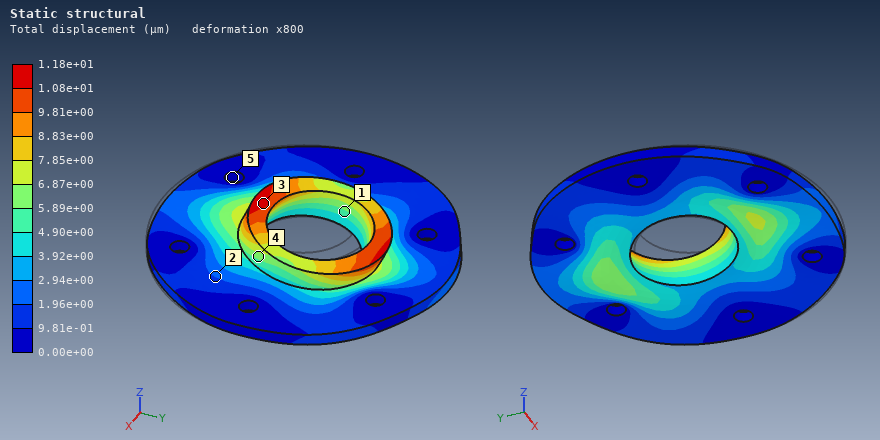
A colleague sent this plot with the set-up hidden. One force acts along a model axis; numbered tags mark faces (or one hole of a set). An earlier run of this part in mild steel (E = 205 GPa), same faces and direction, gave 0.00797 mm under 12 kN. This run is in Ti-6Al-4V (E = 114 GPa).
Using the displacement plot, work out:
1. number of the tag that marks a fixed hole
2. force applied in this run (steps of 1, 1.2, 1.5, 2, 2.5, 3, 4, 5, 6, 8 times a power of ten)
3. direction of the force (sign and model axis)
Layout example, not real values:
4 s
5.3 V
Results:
5
10 kN
+Y
